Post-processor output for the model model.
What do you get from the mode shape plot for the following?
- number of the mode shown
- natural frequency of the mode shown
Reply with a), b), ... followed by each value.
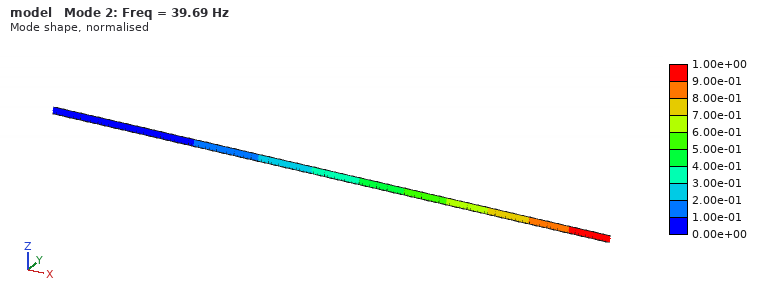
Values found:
a) 2
b) 39.69 Hz
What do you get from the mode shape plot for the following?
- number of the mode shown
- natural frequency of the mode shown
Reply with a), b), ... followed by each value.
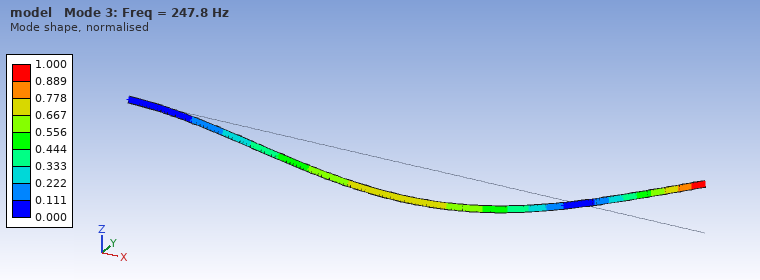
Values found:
a) 3
b) 247.8 Hz
